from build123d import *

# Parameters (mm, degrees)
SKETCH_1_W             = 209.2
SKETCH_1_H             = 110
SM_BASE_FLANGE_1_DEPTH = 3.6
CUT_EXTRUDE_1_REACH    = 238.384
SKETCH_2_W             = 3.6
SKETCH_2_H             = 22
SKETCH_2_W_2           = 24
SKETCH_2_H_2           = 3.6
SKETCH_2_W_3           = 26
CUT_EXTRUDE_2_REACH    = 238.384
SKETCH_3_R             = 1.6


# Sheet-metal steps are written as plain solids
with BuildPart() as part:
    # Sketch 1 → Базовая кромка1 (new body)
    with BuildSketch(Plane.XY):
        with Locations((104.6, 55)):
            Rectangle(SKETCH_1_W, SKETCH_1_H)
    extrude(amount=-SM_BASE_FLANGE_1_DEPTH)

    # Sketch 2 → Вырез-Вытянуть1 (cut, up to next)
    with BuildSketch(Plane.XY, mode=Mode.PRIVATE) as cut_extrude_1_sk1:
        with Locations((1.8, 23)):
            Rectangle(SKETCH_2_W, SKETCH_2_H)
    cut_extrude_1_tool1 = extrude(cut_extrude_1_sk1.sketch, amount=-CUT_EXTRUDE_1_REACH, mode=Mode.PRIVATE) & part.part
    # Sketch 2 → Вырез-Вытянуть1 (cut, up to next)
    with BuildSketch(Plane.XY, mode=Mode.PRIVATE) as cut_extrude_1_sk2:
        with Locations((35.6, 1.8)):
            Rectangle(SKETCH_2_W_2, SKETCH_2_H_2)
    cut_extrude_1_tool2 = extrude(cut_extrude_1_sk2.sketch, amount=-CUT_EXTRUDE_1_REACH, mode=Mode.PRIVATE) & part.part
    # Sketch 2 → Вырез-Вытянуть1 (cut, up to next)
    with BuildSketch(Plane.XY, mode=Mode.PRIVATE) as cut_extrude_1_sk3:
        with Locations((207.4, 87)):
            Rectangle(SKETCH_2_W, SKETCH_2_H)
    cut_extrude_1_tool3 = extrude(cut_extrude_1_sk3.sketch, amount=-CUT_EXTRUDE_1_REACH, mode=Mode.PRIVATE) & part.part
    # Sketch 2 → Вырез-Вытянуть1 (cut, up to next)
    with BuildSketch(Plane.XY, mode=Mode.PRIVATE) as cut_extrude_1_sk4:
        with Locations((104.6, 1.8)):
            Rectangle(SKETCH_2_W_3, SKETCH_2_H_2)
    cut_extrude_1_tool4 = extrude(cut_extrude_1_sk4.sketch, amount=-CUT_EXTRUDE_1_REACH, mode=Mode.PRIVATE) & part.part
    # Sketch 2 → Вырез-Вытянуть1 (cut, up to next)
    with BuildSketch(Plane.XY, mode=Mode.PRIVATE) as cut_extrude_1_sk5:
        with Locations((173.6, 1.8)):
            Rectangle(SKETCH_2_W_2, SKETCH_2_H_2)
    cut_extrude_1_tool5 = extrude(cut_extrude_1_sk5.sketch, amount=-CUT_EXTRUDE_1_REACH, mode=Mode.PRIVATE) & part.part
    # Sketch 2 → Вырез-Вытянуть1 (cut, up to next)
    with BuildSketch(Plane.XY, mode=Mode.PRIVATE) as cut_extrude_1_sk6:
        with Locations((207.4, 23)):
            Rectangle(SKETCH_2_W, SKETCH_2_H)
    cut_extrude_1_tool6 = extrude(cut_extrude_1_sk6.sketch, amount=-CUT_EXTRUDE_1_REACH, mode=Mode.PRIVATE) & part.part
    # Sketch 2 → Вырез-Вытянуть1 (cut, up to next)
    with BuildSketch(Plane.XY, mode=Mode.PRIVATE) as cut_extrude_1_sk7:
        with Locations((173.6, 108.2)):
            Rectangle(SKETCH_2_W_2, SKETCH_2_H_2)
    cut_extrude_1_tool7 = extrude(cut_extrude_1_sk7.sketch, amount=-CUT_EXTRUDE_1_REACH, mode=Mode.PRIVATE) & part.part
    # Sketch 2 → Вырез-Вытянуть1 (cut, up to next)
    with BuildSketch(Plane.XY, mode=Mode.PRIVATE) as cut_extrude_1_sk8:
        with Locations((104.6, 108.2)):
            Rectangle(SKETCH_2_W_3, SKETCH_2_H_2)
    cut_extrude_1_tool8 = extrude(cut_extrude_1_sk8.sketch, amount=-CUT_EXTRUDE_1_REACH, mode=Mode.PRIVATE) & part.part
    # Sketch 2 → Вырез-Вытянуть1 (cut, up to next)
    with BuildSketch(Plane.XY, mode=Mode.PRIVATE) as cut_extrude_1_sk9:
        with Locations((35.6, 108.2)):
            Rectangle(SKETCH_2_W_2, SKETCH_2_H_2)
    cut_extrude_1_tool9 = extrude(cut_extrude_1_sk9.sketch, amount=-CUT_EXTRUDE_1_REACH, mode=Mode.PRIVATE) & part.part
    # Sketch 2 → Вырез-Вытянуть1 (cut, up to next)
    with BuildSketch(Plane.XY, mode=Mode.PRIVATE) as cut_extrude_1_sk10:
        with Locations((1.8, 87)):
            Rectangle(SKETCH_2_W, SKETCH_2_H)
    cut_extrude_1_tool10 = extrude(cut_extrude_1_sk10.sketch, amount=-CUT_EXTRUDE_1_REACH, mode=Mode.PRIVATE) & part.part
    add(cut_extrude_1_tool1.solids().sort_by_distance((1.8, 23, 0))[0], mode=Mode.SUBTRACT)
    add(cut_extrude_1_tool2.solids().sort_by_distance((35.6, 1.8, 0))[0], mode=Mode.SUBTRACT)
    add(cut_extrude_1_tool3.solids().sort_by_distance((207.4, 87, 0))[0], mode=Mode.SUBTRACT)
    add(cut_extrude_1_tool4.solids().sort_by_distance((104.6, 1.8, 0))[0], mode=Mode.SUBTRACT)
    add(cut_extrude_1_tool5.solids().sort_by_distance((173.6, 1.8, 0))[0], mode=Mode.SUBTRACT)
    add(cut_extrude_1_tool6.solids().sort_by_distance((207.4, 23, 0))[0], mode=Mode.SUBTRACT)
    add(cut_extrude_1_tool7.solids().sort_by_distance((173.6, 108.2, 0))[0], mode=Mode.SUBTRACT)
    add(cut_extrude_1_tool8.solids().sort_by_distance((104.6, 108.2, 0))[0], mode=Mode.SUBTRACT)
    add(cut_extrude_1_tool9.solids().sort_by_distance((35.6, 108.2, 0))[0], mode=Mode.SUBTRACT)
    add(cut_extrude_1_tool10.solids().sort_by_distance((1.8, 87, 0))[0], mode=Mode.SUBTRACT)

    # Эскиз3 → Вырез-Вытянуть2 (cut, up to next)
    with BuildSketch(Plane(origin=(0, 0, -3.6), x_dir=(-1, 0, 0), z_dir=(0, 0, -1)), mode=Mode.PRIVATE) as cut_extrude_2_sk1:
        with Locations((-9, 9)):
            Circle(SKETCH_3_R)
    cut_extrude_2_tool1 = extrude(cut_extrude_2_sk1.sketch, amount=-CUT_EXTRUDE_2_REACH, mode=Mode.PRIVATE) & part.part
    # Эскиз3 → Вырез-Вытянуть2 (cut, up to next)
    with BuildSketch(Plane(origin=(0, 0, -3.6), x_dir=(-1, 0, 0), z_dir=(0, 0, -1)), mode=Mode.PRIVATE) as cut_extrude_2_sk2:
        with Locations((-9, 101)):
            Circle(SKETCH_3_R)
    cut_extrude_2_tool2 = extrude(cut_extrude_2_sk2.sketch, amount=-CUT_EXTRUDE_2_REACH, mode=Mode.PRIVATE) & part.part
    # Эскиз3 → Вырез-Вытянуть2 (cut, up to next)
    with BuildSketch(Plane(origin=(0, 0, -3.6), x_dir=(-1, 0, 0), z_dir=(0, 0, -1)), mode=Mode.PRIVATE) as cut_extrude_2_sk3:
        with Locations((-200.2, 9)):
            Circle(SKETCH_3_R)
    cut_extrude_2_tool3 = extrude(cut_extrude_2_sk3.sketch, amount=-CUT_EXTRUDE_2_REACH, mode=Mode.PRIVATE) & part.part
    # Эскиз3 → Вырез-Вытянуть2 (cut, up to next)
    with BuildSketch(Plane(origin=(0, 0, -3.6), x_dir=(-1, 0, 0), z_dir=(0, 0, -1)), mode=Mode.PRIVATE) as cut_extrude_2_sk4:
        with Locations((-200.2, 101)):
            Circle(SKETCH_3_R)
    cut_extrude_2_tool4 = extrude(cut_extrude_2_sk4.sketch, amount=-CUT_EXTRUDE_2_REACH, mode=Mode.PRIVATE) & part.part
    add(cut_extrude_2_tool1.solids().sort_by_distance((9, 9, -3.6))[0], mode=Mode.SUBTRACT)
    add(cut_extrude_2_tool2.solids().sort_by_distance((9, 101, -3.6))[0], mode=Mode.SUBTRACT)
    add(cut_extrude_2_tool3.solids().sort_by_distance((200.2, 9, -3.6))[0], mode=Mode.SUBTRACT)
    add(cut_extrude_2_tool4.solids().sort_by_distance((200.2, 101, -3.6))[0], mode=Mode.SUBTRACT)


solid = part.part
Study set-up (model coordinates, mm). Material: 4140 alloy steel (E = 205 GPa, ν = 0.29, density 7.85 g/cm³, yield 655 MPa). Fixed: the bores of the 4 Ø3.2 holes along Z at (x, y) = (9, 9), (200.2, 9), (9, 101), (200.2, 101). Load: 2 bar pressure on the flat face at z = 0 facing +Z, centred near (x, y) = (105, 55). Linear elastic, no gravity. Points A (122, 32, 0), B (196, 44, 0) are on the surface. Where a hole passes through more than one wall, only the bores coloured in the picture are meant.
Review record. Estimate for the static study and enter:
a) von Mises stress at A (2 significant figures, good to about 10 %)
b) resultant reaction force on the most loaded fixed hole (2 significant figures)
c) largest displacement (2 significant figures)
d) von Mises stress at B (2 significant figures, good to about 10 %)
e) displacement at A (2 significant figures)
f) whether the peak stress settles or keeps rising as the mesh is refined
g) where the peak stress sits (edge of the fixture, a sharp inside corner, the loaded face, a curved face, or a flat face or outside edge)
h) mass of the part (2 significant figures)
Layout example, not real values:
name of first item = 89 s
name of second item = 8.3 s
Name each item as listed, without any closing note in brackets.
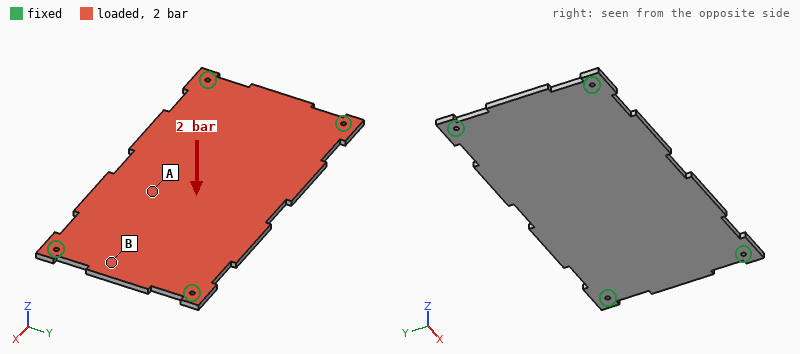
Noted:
von Mises stress at A = 150 MPa
resultant reaction force on the most loaded fixed hole = 1.1 kN
largest displacement = 1.4 mm
von Mises stress at B = 73 MPa
displacement at A = 1.3 mm
whether the peak stress settles or keeps rising as the mesh is refined = keeps rising
where the peak stress sits = edge of the fixture
mass of the part = 630 g
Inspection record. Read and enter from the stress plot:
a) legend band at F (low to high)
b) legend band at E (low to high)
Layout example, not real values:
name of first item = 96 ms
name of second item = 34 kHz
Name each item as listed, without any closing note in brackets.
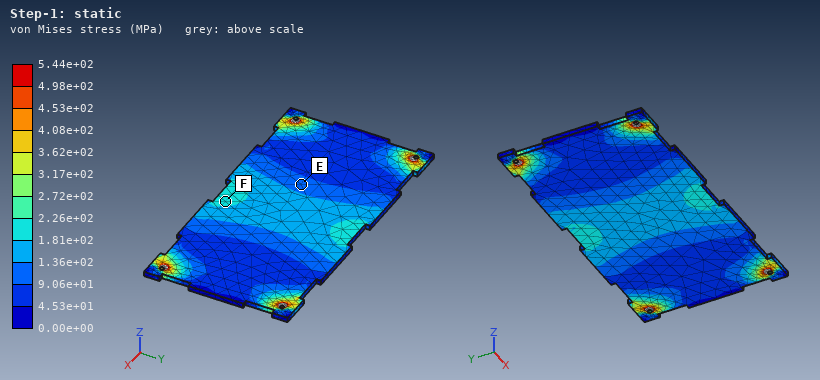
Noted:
legend band at F = 1.81e+02 to 2.26e+02 MPa
legend band at E = 9.06e+01 to 1.36e+02 MPa
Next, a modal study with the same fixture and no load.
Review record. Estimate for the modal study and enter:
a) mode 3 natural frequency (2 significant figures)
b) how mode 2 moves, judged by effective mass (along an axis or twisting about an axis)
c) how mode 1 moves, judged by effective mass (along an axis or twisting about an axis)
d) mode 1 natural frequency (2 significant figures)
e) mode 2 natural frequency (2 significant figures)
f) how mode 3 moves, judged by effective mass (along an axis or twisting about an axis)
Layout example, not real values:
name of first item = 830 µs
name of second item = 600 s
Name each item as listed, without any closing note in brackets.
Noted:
mode 3 natural frequency = 1200 Hz
how mode 2 moves, judged by effective mass = twisting about X
how mode 1 moves, judged by effective mass = along Z
mode 1 natural frequency = 410 Hz
mode 2 natural frequency = 770 Hz
how mode 3 moves, judged by effective mass = twisting about Y
